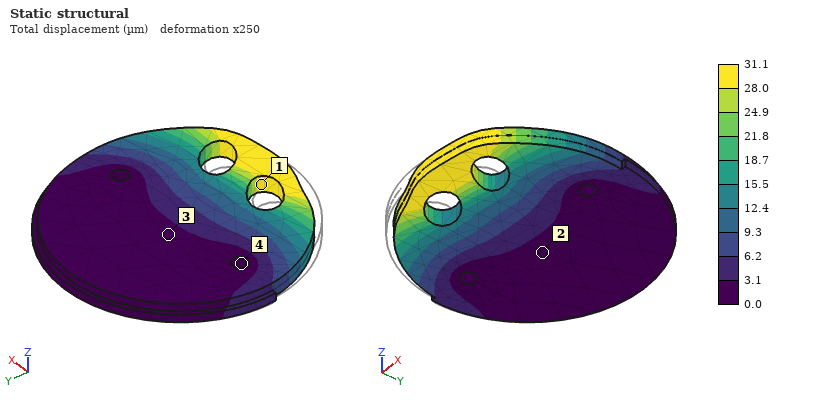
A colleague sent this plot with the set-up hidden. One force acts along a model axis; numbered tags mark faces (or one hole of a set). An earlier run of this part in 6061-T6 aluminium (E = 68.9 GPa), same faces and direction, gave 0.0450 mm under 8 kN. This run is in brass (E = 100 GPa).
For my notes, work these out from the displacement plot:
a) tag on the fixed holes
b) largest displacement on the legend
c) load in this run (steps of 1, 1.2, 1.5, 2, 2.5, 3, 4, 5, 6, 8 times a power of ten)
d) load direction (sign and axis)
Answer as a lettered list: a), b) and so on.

a) 4
b) 31.1 µm
c) 8 kN
d) +X
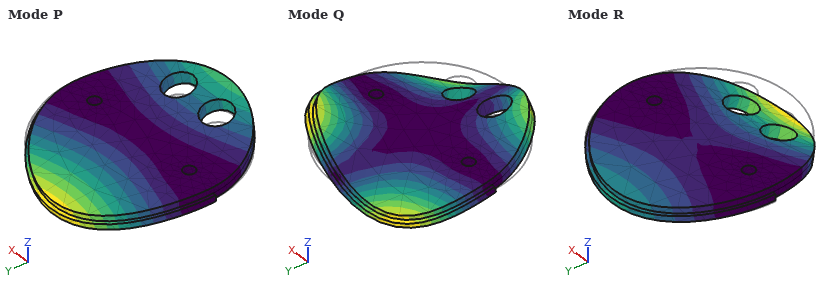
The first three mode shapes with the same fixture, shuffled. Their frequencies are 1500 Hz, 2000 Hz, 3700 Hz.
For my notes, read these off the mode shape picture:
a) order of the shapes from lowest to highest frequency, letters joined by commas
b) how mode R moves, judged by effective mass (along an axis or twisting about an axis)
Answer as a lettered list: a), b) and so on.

a) P, R, Q
b) along Z
